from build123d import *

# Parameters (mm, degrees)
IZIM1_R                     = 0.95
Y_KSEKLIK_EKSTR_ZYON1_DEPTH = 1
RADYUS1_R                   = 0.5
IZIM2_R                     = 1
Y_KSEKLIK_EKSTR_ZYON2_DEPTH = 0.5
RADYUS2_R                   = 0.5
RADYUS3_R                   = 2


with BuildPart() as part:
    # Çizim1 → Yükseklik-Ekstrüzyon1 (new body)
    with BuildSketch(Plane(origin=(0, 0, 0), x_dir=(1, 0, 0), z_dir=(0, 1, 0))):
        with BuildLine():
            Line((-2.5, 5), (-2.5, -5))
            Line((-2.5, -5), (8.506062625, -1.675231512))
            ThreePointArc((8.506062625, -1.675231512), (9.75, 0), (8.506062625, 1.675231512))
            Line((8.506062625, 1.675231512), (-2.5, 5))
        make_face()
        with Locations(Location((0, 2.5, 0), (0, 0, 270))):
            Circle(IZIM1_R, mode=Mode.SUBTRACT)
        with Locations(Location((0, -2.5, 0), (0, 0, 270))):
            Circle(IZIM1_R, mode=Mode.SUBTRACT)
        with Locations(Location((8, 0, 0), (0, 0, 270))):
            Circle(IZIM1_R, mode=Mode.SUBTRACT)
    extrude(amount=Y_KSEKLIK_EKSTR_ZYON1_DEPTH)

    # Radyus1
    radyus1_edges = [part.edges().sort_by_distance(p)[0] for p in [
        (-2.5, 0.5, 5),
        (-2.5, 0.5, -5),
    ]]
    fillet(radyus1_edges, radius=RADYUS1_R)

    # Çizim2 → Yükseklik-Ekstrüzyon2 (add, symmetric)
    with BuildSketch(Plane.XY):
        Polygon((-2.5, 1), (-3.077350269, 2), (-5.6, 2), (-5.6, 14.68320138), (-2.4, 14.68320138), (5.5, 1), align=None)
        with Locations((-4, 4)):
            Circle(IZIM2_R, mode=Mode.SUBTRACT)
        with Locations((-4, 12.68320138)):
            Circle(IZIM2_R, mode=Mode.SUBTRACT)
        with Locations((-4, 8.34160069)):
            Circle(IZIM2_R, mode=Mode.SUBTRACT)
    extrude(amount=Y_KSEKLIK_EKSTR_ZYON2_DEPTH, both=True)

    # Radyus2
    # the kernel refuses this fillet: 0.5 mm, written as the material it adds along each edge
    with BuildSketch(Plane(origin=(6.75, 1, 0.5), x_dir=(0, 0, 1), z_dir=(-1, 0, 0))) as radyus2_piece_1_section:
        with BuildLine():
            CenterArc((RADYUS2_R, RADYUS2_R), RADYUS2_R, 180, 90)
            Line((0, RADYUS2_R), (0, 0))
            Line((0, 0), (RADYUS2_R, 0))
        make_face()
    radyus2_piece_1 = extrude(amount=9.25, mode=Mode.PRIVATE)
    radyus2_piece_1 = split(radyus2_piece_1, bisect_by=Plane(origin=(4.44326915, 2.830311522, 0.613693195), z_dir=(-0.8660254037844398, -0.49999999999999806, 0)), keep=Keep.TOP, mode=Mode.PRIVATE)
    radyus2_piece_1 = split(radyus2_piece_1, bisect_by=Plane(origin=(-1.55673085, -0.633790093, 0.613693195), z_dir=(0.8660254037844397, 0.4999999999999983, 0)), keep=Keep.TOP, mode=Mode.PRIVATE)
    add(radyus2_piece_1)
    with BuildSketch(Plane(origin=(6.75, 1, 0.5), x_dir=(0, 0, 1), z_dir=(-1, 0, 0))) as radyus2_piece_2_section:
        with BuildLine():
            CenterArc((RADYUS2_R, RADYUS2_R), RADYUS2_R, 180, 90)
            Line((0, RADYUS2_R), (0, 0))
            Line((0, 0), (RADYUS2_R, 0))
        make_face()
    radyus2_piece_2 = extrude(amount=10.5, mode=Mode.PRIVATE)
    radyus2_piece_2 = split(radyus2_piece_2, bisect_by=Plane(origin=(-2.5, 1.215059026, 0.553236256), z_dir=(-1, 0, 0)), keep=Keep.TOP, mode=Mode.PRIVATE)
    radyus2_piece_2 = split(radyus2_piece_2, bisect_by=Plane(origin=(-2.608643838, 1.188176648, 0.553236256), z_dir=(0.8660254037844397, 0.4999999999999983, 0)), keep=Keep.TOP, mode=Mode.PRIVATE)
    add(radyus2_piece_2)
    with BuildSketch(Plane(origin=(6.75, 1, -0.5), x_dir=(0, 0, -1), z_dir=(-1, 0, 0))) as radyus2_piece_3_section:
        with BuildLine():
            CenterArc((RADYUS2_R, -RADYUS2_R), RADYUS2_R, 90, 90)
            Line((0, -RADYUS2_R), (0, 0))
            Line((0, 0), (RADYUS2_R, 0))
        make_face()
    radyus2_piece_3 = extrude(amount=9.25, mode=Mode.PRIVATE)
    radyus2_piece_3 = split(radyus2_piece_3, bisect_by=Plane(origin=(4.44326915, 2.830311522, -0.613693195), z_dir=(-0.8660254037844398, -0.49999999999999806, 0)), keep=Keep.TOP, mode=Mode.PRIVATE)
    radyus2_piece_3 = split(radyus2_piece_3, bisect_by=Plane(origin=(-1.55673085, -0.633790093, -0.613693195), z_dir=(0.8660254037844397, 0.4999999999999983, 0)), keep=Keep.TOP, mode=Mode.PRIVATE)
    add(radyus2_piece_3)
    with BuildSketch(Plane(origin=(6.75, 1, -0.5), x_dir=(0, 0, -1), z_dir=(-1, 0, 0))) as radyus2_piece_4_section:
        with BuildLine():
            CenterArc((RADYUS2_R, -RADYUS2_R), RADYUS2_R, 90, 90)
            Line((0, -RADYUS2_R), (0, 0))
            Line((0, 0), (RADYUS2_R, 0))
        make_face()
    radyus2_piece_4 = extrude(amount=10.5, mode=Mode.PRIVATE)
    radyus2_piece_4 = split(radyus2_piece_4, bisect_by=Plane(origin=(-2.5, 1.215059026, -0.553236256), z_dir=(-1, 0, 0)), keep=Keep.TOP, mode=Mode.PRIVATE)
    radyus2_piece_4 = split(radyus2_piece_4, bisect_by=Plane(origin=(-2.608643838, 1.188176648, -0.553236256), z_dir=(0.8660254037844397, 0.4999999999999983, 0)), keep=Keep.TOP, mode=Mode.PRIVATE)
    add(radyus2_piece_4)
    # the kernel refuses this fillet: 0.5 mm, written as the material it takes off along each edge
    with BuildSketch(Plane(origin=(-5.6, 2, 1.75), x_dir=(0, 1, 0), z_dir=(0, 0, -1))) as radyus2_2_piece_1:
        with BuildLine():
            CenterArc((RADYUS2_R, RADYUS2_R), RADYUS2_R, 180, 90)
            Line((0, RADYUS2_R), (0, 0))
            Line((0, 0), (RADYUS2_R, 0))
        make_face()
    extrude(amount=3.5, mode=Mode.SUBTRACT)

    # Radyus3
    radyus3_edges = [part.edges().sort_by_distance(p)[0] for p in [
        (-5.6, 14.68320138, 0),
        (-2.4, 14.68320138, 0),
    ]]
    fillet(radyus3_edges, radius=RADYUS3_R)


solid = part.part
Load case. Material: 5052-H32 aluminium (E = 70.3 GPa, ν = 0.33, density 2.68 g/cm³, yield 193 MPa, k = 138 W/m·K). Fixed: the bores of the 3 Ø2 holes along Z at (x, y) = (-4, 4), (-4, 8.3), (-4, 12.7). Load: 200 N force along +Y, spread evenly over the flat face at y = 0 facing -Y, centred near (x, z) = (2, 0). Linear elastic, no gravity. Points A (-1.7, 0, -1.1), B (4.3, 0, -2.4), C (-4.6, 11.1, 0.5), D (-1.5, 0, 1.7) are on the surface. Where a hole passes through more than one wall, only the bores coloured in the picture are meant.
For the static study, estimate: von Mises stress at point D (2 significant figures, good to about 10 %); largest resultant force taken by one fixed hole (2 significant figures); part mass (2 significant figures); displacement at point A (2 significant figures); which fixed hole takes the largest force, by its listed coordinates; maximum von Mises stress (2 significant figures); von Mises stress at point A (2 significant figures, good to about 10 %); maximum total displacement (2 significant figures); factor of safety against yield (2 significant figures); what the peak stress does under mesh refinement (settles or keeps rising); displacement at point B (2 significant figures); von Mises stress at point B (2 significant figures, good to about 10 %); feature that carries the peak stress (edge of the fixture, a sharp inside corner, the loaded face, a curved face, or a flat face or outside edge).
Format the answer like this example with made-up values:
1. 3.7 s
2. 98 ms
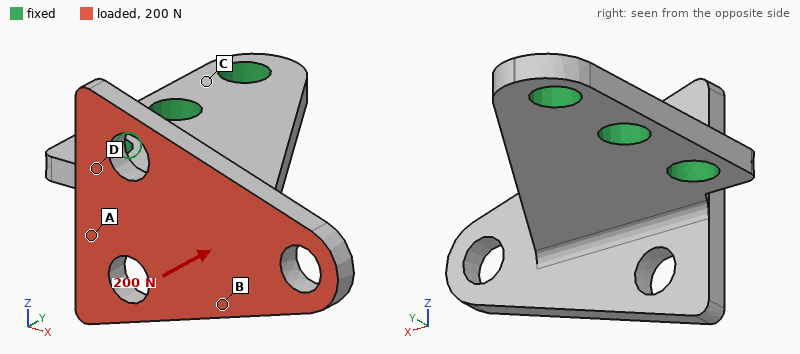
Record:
1. 68 MPa
2. 160 N
3. 0.41 g
4. 9.4 µm
5. (-4, 4)
6. 180 MPa
7. 79 MPa
8. 55 µm
9. 1.1
10. settles
11. 21 µm
12. 50 MPa
13. a curved face
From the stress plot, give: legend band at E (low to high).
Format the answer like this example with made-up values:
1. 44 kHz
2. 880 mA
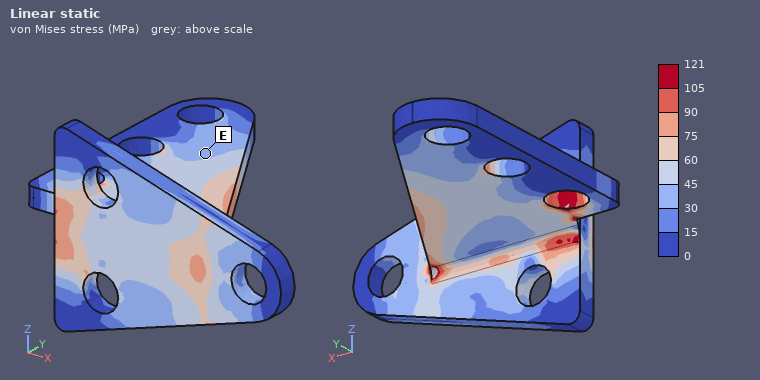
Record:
1. 30 to 45 MPa
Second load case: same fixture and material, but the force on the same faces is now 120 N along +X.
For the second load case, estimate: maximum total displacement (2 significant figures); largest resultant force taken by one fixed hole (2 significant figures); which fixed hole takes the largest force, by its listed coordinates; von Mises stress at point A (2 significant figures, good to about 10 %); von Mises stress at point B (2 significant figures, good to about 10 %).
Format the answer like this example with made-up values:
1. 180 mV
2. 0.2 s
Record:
1. 23 µm
2. 180 N
3. (-4, 4)
4. 13 MPa
5. 13 MPa
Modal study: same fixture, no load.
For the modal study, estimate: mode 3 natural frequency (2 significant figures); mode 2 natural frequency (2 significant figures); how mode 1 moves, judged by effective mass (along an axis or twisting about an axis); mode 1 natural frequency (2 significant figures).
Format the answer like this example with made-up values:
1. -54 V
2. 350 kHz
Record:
1. 29 kHz
2. 17 kHz
3. along Z
4. 5900 Hz
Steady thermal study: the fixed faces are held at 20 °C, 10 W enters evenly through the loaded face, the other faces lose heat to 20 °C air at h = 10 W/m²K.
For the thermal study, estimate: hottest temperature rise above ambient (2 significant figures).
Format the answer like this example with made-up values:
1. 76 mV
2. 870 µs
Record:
1. 79 K
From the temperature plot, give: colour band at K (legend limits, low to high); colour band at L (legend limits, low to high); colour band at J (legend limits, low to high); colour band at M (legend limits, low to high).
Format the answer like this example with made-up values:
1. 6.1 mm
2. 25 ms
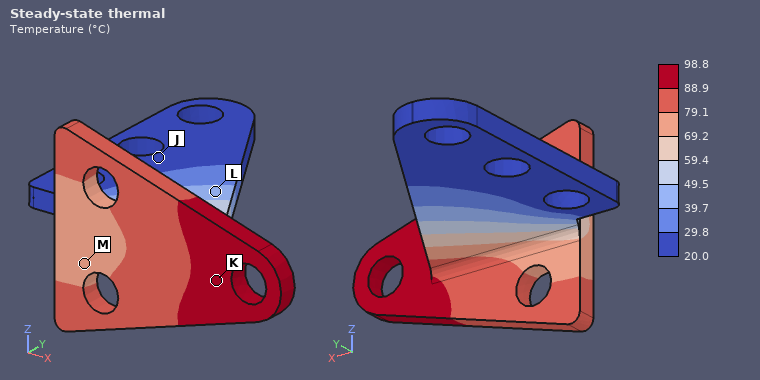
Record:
1. 88.9 to 98.8 °C
2. 39.7 to 49.5 °C
3. 20.0 to 29.8 °C
4. 69.2 to 79.1 °C
